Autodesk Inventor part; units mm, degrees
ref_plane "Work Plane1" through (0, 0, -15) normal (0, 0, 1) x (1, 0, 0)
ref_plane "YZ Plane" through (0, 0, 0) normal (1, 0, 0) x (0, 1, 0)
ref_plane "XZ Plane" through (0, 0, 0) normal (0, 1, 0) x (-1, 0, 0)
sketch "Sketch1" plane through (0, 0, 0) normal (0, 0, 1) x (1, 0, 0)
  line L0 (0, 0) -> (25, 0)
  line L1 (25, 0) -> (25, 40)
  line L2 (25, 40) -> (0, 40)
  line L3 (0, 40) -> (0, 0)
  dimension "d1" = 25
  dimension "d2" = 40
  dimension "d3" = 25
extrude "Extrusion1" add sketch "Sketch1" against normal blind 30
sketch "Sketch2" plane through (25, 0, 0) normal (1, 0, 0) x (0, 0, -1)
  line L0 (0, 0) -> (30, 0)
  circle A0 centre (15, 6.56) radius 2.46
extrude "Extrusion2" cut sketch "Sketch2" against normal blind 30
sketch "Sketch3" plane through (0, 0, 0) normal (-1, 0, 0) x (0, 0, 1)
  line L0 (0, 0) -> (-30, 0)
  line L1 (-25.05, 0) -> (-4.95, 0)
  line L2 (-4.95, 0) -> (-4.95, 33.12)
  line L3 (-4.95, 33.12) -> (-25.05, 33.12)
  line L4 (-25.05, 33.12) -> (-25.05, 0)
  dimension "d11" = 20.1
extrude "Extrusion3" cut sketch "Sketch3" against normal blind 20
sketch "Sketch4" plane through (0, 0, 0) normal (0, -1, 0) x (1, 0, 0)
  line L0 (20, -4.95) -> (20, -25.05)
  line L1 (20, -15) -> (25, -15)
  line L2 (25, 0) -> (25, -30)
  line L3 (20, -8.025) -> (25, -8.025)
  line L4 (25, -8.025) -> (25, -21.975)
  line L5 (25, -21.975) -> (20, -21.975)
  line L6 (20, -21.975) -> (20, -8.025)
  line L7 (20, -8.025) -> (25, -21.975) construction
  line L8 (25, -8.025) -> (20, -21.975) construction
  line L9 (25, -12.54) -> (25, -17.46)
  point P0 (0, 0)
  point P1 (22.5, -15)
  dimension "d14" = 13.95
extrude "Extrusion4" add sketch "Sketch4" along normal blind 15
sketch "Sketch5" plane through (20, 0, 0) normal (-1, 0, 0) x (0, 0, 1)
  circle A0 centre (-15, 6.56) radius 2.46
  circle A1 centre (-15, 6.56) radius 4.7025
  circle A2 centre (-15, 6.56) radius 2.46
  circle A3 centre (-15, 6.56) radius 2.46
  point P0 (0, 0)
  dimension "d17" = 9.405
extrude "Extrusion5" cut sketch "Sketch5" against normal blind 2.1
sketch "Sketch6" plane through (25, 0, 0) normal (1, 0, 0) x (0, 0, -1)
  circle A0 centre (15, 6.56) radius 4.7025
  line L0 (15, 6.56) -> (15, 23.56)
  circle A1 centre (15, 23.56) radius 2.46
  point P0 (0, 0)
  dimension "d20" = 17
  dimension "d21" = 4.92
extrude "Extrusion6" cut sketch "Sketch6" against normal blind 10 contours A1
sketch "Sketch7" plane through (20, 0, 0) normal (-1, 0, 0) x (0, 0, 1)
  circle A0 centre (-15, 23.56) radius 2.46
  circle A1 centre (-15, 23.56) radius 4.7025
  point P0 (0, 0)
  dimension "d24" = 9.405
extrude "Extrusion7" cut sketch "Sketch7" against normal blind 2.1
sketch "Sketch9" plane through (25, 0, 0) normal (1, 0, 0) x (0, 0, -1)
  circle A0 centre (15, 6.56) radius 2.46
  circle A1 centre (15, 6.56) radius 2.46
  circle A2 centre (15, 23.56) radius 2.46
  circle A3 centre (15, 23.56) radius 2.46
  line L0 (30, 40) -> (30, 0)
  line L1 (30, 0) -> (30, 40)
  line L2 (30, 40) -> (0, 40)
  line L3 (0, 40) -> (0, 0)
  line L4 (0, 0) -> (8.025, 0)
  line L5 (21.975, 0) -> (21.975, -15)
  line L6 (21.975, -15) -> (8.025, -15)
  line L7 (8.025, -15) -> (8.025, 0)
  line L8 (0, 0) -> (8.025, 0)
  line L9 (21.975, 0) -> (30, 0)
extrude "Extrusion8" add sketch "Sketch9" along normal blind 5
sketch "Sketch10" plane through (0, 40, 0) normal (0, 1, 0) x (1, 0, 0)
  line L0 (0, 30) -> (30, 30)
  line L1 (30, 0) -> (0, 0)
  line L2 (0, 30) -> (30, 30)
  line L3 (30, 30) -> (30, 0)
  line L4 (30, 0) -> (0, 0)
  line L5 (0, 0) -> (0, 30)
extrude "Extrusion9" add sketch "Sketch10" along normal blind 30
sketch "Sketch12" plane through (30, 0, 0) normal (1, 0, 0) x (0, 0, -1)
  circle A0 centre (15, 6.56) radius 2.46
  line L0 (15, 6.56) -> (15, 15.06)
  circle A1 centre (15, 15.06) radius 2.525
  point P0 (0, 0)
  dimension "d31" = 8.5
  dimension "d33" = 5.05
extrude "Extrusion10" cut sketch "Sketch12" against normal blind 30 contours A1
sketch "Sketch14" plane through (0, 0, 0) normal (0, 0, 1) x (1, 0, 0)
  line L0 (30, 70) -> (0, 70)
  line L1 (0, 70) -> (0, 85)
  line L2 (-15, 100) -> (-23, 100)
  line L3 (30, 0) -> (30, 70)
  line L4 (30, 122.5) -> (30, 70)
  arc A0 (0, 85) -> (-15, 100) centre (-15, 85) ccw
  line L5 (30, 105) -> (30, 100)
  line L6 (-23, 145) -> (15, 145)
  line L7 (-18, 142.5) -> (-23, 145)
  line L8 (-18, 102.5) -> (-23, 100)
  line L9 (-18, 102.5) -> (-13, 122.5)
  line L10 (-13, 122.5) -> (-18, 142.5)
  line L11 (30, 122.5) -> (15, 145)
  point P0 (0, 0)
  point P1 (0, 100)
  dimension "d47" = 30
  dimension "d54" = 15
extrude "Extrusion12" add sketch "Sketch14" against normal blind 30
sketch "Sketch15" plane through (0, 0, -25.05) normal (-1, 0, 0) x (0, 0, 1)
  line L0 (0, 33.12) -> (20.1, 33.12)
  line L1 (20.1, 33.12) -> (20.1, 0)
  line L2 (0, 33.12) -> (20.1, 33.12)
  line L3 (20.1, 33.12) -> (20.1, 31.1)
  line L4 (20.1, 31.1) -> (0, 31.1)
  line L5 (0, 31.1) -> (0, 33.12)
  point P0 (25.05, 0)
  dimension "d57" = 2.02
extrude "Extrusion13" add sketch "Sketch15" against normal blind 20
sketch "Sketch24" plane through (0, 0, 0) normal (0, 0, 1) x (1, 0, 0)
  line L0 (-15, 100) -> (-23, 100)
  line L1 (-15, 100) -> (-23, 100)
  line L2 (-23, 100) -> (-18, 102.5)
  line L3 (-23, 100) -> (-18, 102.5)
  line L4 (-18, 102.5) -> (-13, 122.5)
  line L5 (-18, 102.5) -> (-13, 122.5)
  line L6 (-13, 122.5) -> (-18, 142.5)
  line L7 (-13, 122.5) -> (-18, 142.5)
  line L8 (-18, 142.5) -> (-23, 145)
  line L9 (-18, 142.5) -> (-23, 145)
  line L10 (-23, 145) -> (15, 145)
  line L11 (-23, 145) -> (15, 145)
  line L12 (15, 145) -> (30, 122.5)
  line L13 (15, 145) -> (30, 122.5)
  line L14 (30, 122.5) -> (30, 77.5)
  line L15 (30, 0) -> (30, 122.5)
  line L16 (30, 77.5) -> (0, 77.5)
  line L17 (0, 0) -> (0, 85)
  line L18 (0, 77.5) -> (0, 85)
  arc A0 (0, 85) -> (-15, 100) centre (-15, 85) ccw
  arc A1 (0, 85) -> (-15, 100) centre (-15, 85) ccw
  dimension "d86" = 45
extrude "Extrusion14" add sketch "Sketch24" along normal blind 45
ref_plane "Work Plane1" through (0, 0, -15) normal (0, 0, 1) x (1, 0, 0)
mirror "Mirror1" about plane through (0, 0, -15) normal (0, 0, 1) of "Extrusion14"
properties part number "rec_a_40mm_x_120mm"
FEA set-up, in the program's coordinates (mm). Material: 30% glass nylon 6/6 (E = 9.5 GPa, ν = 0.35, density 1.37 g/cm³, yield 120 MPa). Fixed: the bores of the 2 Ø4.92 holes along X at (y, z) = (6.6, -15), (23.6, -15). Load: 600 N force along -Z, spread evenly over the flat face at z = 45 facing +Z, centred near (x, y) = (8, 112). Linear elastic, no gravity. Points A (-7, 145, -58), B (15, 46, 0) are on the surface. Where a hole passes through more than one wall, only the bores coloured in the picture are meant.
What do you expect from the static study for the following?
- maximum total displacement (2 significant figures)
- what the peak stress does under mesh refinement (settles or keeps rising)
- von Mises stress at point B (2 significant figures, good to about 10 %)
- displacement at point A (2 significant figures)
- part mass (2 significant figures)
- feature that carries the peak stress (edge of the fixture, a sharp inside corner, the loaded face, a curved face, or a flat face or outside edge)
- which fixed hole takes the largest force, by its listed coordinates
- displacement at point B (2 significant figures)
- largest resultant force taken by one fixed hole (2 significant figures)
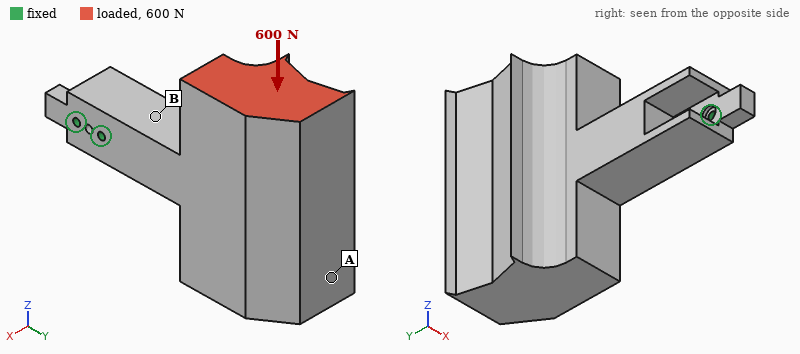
1.2 mm
keeps rising
9.6 MPa
1.1 mm
510 g
edge of the fixture
(23.6, -15)
0.19 mm
2.9 kN
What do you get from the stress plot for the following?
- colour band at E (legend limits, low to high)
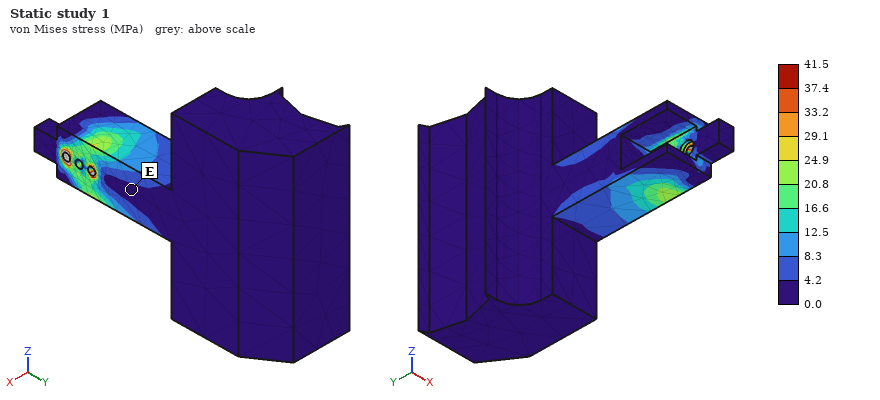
0.0 to 4.2 MPa
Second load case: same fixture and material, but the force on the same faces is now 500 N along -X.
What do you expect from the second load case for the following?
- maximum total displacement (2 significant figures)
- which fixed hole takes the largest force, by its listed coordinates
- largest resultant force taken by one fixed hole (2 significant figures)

2.1 mm
(23.6, -15)
2.3 kN
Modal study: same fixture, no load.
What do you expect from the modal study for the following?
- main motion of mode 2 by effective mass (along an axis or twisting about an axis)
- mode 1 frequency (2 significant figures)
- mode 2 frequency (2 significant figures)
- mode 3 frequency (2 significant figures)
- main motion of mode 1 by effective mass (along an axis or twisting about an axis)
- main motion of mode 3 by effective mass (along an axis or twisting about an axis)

along Z
180 Hz
200 Hz
300 Hz
along X
twisting about Y
